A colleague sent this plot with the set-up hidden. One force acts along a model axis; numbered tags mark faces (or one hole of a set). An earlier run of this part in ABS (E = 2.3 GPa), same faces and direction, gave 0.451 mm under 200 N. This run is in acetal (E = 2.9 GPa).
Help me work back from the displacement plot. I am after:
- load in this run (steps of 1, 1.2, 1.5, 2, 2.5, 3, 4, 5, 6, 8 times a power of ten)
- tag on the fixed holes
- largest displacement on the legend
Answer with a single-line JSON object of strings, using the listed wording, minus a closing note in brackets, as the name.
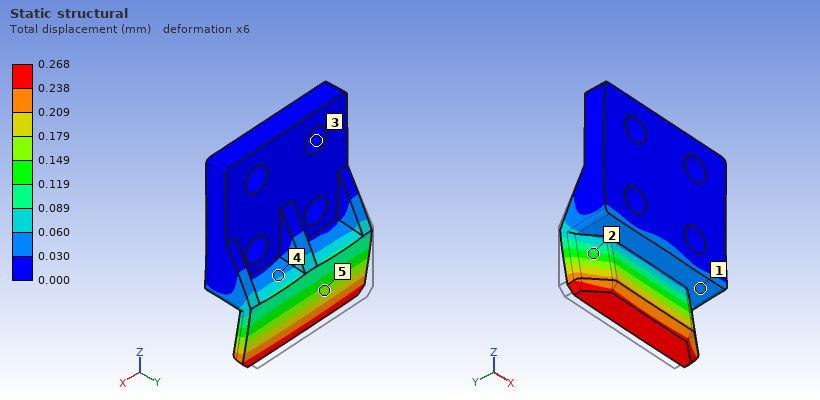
{"load in this run": "150 N", "tag on the fixed holes": "3", "largest displacement on the legend": "0.268 mm"}
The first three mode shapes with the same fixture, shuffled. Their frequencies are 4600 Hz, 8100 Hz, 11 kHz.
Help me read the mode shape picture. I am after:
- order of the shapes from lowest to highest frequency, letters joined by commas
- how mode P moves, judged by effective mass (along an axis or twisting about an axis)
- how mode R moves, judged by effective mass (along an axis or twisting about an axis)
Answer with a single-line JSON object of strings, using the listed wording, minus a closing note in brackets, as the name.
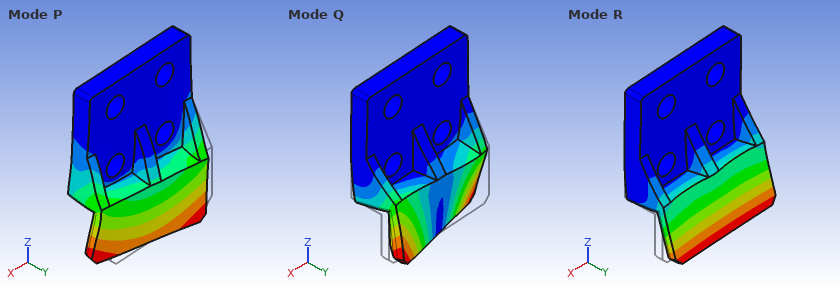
{"order of the shapes from lowest to highest frequency, letters joined by commas": "R, Q, P", "how mode P moves, judged by effective mass": "along X", "how mode R moves, judged by effective mass": "along Y"}
